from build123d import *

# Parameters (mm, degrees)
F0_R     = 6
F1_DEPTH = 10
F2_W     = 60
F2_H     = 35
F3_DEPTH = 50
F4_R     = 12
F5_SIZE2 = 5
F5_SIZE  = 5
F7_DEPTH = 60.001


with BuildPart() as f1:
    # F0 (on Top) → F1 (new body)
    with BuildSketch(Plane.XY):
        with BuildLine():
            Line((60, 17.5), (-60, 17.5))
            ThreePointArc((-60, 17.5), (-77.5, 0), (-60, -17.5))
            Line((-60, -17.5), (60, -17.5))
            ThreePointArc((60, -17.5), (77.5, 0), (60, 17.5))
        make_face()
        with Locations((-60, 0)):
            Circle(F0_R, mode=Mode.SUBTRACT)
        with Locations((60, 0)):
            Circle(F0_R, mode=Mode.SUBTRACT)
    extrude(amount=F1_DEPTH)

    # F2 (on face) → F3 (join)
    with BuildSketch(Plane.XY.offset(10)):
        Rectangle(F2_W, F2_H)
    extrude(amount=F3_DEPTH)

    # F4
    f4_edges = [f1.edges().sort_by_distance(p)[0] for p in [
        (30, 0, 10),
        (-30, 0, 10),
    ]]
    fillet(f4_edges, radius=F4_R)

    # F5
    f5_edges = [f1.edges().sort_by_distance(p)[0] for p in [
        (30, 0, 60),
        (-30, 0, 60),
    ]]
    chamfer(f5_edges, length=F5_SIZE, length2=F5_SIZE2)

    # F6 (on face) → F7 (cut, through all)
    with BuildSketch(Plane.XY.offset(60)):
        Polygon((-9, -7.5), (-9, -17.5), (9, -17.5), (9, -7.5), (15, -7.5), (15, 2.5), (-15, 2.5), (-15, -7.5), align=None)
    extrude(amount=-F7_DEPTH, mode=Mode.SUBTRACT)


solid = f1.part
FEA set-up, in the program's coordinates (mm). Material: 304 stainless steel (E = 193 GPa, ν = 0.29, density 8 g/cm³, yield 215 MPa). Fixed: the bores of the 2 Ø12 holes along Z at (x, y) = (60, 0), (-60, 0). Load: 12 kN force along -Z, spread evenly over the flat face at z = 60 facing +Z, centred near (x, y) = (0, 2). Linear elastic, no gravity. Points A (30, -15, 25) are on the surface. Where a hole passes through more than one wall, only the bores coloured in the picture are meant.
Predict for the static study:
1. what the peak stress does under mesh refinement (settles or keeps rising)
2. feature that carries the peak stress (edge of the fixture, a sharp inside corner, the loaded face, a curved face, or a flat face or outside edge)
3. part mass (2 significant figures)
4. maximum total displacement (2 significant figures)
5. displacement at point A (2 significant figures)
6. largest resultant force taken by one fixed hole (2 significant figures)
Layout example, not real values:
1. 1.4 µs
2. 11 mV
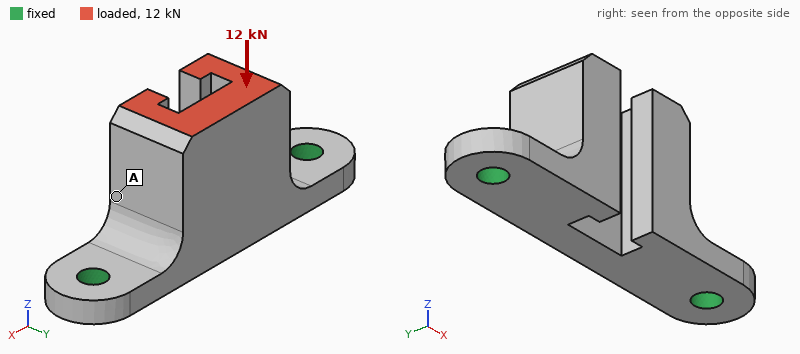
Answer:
1. keeps rising
2. edge of the fixture
3. 1.0 kg
4. 44 µm
5. 25 µm
6. 7.1 kN
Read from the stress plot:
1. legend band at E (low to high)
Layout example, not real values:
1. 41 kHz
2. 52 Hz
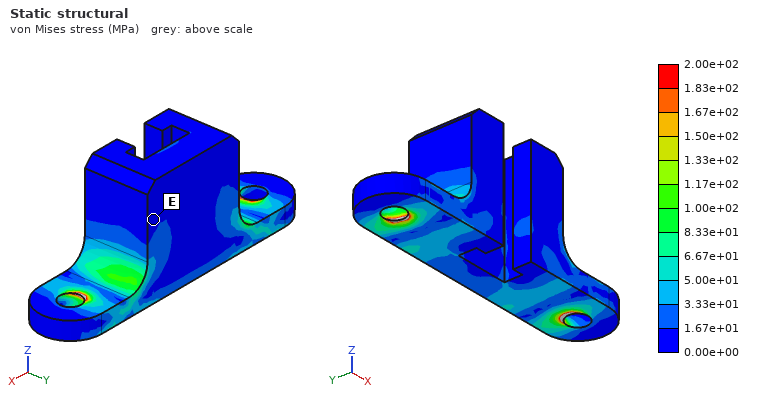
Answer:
1. 0.00e+00 to 1.67e+01 MPa
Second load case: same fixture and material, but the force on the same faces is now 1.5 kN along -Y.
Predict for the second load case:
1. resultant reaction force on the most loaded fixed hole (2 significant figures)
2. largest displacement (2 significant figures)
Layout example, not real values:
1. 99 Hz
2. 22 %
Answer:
1. 890 N
2. 69 µm
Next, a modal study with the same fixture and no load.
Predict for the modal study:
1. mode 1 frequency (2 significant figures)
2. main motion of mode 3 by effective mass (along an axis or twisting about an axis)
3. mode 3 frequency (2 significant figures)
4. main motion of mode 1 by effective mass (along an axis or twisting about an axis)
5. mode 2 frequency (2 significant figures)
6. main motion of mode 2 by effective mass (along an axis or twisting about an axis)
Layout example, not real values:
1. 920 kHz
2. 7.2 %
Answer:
1. 1500 Hz
2. along X
3. 4500 Hz
4. along Y
5. 3500 Hz
6. along Z
